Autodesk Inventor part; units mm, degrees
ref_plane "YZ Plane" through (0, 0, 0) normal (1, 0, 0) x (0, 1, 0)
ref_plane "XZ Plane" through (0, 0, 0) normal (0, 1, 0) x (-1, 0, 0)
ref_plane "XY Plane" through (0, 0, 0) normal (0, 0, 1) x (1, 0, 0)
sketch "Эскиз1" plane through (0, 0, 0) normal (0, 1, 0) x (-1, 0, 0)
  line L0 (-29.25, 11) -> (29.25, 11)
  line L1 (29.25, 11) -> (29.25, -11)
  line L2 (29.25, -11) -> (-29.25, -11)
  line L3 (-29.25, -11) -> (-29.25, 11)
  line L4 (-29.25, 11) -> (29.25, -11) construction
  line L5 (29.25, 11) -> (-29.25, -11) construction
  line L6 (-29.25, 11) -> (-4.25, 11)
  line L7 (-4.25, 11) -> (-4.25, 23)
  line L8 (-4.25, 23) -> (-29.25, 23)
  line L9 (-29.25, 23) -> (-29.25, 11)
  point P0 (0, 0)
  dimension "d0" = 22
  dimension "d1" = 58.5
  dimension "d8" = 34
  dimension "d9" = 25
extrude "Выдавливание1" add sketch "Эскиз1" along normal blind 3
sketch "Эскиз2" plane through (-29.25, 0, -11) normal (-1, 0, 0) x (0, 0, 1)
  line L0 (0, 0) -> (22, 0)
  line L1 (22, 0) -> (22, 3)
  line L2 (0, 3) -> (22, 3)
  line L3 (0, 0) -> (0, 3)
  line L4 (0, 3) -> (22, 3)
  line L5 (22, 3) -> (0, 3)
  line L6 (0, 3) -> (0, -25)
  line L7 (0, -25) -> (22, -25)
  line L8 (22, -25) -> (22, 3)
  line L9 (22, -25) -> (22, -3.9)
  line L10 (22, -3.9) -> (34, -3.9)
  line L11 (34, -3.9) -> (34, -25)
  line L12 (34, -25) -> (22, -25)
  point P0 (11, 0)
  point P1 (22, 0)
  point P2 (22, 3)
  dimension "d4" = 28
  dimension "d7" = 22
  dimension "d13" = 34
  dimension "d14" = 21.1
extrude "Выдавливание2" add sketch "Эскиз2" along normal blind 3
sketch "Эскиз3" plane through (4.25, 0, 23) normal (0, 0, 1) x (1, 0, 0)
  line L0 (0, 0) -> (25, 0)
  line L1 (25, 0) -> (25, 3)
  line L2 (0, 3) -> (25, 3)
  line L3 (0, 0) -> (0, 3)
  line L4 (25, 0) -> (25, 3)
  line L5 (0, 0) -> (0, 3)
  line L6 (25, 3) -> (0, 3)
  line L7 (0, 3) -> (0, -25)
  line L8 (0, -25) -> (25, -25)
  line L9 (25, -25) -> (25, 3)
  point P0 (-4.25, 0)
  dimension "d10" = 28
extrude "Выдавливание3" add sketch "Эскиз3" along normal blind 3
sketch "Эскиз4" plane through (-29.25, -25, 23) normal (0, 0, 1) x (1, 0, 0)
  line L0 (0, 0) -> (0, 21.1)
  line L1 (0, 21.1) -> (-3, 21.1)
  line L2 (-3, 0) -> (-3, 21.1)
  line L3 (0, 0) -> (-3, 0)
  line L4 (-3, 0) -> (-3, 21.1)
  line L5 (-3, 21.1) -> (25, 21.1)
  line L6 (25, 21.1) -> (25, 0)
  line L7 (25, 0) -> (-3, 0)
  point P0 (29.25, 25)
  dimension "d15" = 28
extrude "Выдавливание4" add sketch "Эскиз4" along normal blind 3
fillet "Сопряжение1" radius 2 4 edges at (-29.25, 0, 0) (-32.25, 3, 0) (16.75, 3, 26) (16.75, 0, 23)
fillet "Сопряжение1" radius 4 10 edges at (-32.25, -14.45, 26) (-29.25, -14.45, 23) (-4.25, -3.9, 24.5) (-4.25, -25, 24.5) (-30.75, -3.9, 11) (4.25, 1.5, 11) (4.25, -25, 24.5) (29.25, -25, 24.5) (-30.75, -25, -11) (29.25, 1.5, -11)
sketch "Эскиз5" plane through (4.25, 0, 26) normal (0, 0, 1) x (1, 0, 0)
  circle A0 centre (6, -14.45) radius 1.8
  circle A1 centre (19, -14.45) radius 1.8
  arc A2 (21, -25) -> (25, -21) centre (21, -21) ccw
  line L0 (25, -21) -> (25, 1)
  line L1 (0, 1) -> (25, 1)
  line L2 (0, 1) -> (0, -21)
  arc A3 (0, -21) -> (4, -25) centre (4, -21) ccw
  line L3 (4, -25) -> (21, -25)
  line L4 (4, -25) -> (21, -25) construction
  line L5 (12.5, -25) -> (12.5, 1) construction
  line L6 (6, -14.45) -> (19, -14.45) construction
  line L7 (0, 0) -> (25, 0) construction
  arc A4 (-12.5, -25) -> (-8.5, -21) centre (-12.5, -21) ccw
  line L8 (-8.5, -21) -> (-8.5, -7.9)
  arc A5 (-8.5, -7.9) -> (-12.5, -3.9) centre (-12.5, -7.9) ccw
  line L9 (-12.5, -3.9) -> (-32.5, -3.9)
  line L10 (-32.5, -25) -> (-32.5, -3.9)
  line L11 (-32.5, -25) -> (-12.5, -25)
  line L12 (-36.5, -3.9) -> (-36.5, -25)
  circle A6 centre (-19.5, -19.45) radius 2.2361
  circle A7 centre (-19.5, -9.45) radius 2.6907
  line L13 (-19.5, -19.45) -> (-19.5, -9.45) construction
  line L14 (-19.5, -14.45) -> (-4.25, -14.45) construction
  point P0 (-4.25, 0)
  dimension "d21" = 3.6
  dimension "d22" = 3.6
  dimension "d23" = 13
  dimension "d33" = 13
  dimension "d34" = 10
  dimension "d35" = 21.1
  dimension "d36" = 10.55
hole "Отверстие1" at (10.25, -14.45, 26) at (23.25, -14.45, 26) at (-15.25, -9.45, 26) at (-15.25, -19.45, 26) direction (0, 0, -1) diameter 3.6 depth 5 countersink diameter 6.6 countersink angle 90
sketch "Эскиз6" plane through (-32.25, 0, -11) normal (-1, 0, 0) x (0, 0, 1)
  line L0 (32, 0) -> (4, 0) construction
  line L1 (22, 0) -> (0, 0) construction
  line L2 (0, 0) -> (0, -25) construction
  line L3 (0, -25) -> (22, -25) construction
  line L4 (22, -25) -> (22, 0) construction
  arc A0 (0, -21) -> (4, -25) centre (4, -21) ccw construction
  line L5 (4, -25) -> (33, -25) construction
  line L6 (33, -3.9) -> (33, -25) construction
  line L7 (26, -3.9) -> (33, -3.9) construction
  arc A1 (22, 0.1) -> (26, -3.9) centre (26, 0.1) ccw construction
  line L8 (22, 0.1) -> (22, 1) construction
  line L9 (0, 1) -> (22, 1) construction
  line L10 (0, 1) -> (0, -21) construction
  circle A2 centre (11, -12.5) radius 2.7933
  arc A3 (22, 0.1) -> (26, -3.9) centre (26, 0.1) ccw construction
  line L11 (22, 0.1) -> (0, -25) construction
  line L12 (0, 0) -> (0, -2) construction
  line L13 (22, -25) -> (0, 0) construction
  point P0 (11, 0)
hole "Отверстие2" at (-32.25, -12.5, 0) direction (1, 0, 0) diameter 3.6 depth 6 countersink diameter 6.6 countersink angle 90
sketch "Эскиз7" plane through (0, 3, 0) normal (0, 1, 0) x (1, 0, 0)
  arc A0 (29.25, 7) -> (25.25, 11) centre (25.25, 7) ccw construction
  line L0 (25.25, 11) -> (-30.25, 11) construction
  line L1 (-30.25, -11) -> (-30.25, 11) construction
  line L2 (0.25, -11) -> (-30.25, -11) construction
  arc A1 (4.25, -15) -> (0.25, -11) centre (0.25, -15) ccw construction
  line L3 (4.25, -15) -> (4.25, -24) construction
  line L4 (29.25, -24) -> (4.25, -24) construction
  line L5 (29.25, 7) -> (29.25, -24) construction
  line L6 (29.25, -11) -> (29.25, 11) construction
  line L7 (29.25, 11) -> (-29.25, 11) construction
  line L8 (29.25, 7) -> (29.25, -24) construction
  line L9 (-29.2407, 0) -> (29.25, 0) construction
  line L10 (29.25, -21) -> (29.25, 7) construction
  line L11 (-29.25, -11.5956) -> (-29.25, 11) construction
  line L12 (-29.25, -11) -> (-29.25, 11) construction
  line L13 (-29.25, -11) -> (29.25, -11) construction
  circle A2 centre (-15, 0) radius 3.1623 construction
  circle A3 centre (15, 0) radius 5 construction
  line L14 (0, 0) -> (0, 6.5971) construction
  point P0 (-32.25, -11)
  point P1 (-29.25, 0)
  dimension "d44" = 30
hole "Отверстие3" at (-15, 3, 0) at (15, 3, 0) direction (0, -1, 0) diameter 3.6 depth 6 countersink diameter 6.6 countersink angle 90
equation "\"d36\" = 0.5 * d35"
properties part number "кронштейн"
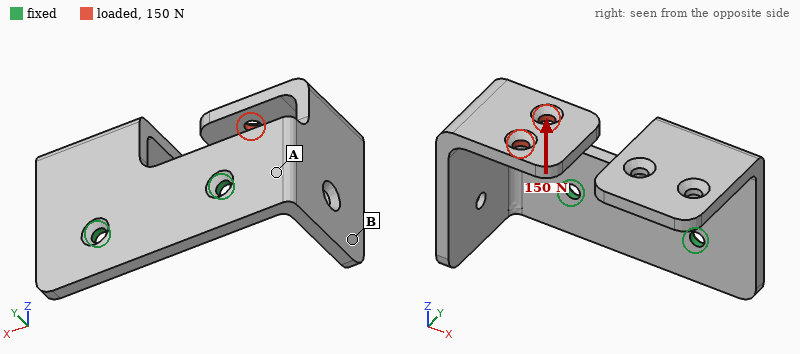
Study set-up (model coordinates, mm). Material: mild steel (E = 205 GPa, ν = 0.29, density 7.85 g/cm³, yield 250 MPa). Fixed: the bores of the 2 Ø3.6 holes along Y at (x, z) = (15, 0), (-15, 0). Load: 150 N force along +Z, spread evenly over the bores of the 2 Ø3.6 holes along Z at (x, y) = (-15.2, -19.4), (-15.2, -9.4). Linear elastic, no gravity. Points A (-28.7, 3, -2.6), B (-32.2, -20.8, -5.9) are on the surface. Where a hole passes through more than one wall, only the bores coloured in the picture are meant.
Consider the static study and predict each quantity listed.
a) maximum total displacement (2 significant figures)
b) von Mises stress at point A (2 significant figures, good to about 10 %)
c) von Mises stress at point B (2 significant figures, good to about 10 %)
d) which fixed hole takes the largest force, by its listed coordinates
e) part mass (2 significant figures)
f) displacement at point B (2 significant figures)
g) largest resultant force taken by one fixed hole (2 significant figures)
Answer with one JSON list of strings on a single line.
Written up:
["0.26 mm", "56 MPa", "17 MPa", "(-15, 0)", "85 g", "0.068 mm", "160 N"]
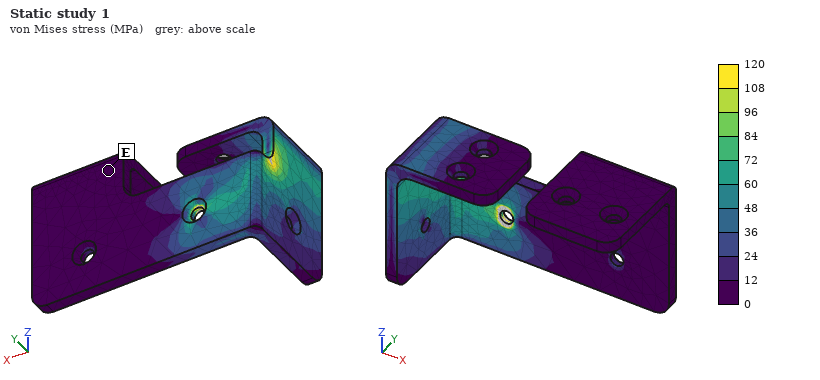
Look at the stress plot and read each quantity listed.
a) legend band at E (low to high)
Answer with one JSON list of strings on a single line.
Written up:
["0 to 12 MPa"]
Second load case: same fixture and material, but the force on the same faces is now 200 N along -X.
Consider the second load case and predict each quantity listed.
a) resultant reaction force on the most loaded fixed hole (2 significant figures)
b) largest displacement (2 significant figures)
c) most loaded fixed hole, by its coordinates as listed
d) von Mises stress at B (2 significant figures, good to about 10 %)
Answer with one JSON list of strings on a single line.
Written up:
["390 N", "0.37 mm", "(-15, 0)", "35 MPa"]
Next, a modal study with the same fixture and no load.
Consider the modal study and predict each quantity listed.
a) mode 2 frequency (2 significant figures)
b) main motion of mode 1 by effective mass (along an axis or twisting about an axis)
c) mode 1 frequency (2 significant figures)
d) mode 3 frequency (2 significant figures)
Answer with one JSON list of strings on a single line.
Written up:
["1000 Hz", "along X", "920 Hz", "1200 Hz"]
